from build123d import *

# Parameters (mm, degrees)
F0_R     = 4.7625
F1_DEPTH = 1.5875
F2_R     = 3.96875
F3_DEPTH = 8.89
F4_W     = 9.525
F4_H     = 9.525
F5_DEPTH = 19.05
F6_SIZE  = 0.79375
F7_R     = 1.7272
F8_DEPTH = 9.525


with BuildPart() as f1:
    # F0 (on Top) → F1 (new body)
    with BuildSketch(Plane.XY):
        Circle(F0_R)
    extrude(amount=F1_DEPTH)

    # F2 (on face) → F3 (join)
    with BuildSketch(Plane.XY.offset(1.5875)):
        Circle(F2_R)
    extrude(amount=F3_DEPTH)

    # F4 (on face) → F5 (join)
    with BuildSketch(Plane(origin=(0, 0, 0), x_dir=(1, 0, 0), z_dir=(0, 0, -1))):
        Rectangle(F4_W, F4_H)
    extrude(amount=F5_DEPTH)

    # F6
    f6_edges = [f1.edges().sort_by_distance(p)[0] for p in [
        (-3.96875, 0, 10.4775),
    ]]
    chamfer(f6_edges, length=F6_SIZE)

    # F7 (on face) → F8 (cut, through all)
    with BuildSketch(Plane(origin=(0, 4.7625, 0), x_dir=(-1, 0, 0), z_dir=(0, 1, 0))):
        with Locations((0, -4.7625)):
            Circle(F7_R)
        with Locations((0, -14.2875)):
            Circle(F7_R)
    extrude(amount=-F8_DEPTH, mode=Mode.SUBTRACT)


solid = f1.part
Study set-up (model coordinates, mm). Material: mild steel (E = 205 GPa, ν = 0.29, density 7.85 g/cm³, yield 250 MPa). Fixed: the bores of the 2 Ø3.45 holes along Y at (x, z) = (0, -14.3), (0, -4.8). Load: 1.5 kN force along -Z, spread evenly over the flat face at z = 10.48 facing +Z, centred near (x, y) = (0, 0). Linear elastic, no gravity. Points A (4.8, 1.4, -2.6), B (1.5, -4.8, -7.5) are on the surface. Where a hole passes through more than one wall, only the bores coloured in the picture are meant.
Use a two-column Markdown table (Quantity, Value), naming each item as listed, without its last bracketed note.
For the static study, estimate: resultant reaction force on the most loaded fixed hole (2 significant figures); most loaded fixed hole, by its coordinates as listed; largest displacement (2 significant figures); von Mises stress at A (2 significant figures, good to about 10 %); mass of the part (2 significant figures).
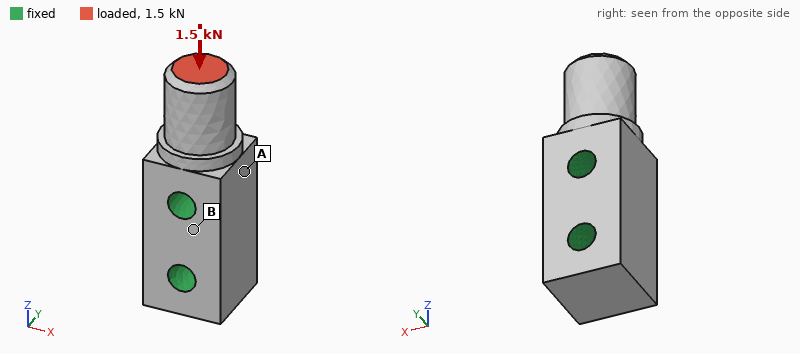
| Quantity | Value |
|---|---|
| resultant reaction force on the most loaded fixed hole | 1.4 kN |
| most loaded fixed hole, by its coordinates as listed | (0, -4.8) |
| largest displacement | 2.2 µm |
| von Mises stress at A | 10 MPa |
| mass of the part | 16 g |
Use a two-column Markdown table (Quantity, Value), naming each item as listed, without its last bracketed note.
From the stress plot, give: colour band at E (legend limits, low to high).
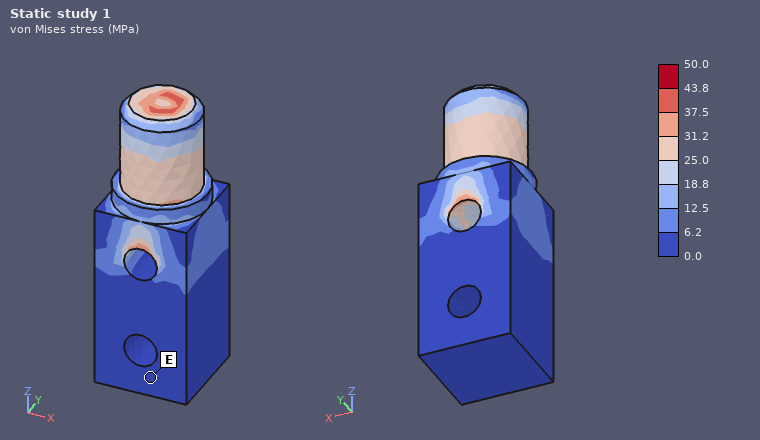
| Quantity | Value |
|---|---|
| colour band at E | 0.0 to 6.2 MPa |
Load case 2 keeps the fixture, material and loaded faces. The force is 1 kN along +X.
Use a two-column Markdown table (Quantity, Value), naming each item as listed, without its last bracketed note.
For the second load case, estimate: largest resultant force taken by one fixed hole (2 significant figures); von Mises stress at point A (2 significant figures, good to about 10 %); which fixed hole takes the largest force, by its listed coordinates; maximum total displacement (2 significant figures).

| Quantity | Value |
|---|---|
| largest resultant force taken by one fixed hole | 1.6 kN |
| von Mises stress at point A | 95 MPa |
| which fixed hole takes the largest force, by its listed coordinates | (0, -4.8) |
| maximum total displacement | 22 µm |
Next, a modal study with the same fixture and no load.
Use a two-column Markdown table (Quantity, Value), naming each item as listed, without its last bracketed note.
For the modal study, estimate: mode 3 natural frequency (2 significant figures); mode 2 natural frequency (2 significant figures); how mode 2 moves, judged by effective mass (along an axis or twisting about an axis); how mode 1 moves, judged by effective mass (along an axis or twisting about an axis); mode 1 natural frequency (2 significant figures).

| Quantity | Value |
|---|---|
| mode 3 natural frequency | 69 kHz |
| mode 2 natural frequency | 33 kHz |
| how mode 2 moves, judged by effective mass | along Y |
| how mode 1 moves, judged by effective mass | along X |
| mode 1 natural frequency | 29 kHz |
